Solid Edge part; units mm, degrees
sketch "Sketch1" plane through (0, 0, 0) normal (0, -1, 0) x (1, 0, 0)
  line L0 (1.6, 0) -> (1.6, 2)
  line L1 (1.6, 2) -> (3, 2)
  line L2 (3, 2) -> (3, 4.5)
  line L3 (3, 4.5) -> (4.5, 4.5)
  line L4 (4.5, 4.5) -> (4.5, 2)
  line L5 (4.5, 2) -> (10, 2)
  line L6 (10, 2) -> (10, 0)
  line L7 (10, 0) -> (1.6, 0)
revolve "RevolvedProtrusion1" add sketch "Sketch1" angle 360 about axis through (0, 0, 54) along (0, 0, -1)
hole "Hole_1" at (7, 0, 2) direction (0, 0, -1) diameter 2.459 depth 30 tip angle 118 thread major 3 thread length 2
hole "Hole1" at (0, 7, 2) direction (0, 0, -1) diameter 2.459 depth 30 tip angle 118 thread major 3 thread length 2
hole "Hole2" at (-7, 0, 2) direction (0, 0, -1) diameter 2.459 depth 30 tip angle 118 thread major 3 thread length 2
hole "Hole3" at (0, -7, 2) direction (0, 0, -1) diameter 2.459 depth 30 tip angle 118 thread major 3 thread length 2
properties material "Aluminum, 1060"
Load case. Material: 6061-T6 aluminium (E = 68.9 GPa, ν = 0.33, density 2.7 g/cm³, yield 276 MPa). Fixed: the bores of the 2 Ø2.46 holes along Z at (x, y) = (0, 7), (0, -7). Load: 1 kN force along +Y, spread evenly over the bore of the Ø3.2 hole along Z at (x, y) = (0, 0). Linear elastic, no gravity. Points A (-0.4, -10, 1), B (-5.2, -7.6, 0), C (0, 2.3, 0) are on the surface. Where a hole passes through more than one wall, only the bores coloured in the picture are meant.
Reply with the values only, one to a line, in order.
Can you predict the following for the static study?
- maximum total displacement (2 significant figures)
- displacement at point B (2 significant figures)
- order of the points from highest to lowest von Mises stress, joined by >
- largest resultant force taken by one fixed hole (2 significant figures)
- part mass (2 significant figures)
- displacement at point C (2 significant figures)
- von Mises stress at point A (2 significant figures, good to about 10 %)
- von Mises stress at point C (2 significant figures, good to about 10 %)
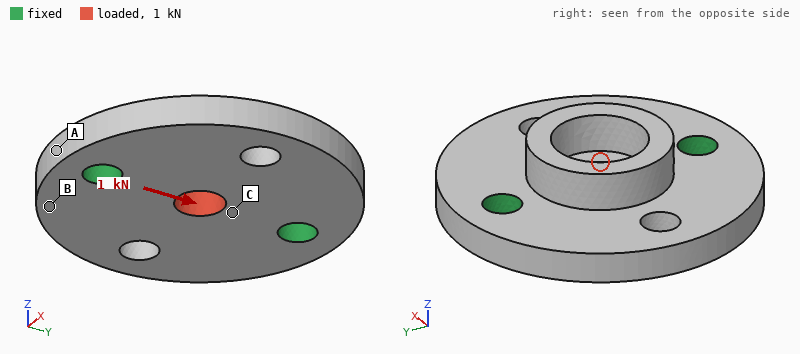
3.8 µm
1.6 µm
C > A > B
500 N
1.8 g
2.9 µm
17 MPa
55 MPa
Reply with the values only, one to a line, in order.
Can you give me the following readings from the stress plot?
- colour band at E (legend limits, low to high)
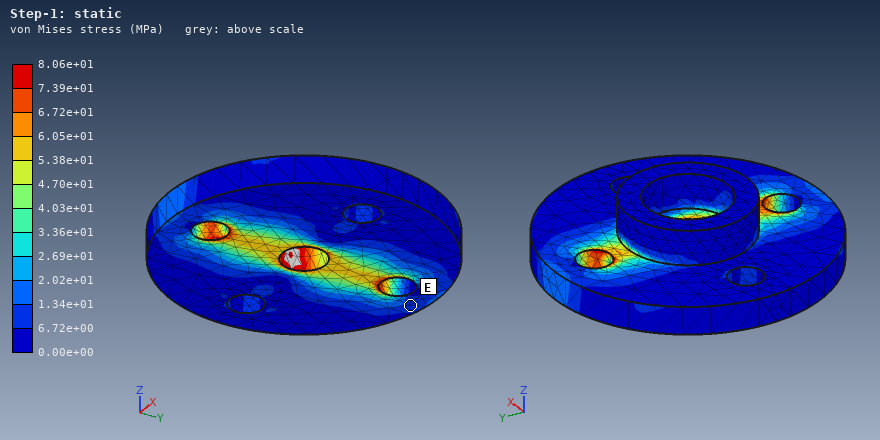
6.72e+00 to 1.34e+01 MPa
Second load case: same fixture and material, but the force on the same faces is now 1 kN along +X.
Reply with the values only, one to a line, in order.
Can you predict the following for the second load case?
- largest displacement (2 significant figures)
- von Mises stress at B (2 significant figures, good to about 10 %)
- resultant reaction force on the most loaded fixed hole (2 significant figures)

6.1 µm
12 MPa
500 N
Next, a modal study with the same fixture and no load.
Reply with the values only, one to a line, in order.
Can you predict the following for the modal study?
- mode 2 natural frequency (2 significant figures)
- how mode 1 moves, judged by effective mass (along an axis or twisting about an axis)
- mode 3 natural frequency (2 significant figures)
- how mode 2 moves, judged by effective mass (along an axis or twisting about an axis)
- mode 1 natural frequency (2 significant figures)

25 kHz
twisting about Y
45 kHz
along Z
19 kHz
